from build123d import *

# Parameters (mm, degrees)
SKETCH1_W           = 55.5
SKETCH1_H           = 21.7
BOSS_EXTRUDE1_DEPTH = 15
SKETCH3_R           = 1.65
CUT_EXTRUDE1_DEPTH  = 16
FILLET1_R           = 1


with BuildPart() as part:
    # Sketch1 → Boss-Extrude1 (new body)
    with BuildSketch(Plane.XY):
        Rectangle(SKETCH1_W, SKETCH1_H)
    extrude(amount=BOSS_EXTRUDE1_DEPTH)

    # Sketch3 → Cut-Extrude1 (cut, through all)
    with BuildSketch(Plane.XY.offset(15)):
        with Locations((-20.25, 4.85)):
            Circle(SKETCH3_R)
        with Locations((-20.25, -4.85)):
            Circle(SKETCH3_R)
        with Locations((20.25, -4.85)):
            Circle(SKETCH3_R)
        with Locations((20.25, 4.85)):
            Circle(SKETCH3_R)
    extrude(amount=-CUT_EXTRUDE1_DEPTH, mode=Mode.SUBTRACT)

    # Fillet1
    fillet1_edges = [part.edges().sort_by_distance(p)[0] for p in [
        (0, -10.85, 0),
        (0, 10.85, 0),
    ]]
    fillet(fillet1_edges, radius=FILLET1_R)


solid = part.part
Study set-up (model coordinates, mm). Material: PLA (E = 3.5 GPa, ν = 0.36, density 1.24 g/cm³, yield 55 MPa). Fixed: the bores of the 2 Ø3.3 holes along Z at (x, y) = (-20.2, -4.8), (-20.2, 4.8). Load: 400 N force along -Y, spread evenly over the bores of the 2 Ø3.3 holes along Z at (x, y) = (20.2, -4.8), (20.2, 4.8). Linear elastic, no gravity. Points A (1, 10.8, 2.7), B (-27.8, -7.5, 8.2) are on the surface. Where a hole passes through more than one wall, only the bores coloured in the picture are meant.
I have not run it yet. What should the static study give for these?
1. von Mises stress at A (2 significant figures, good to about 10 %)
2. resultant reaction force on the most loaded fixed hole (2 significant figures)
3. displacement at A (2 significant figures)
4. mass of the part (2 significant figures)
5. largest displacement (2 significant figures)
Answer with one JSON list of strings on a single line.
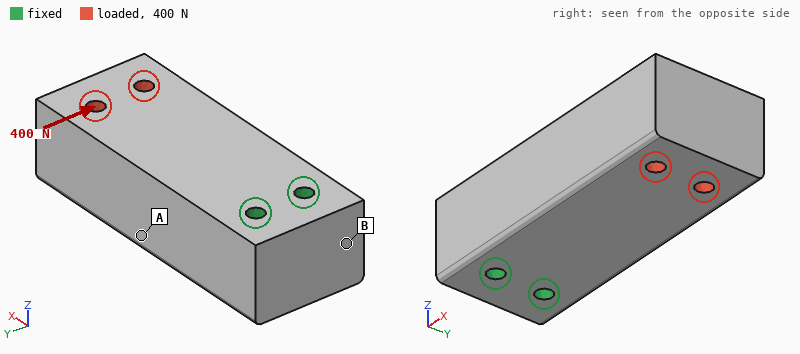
["6.6 MPa", "1.4 kN", "0.14 mm", "22 g", "0.36 mm"]
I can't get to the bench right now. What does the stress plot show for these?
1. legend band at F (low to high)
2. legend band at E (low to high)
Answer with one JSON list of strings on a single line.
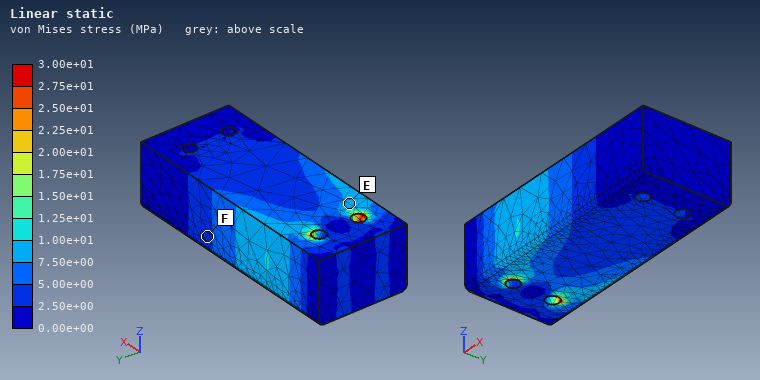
["2.50e+00 to 5.00e+00 MPa", "7.50e+00 to 1.00e+01 MPa"]
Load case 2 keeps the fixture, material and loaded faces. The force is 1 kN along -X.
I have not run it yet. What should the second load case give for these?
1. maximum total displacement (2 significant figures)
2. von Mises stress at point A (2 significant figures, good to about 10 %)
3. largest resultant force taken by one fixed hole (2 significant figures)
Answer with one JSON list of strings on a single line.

["40 µm", "3.1 MPa", "510 N"]
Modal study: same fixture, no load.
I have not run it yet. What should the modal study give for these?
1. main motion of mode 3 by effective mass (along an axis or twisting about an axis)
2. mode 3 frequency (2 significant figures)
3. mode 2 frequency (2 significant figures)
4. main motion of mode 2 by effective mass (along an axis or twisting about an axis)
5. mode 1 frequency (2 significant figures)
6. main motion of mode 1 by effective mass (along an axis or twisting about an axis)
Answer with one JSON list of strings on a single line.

["twisting about X", "4700 Hz", "2100 Hz", "along Y", "1700 Hz", "along Z"]
